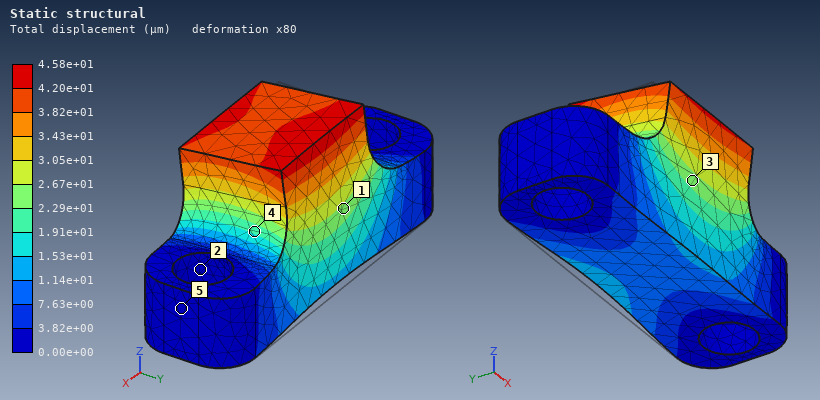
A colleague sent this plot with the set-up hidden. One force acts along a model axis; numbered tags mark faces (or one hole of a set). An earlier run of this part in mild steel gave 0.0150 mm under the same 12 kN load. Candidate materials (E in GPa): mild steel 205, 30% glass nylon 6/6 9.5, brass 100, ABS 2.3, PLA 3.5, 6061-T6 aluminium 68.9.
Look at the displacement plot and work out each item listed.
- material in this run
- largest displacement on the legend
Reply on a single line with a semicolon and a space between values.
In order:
6061-T6 aluminium; 4.58e+01 µm
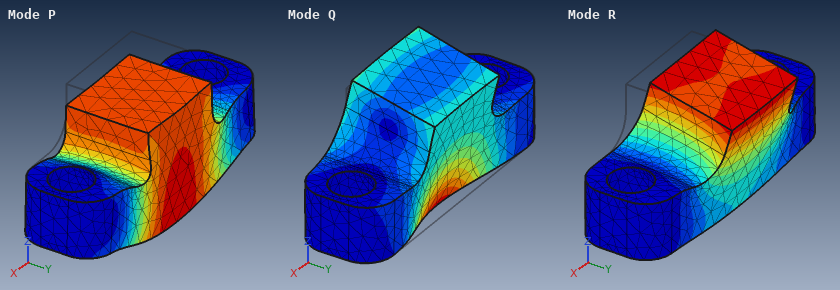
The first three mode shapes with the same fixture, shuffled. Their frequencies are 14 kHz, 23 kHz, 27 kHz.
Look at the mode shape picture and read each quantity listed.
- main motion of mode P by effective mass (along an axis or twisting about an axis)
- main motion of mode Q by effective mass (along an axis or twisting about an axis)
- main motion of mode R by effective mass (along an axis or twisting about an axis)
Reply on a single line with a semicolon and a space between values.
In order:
along Z; along Y; along Y
